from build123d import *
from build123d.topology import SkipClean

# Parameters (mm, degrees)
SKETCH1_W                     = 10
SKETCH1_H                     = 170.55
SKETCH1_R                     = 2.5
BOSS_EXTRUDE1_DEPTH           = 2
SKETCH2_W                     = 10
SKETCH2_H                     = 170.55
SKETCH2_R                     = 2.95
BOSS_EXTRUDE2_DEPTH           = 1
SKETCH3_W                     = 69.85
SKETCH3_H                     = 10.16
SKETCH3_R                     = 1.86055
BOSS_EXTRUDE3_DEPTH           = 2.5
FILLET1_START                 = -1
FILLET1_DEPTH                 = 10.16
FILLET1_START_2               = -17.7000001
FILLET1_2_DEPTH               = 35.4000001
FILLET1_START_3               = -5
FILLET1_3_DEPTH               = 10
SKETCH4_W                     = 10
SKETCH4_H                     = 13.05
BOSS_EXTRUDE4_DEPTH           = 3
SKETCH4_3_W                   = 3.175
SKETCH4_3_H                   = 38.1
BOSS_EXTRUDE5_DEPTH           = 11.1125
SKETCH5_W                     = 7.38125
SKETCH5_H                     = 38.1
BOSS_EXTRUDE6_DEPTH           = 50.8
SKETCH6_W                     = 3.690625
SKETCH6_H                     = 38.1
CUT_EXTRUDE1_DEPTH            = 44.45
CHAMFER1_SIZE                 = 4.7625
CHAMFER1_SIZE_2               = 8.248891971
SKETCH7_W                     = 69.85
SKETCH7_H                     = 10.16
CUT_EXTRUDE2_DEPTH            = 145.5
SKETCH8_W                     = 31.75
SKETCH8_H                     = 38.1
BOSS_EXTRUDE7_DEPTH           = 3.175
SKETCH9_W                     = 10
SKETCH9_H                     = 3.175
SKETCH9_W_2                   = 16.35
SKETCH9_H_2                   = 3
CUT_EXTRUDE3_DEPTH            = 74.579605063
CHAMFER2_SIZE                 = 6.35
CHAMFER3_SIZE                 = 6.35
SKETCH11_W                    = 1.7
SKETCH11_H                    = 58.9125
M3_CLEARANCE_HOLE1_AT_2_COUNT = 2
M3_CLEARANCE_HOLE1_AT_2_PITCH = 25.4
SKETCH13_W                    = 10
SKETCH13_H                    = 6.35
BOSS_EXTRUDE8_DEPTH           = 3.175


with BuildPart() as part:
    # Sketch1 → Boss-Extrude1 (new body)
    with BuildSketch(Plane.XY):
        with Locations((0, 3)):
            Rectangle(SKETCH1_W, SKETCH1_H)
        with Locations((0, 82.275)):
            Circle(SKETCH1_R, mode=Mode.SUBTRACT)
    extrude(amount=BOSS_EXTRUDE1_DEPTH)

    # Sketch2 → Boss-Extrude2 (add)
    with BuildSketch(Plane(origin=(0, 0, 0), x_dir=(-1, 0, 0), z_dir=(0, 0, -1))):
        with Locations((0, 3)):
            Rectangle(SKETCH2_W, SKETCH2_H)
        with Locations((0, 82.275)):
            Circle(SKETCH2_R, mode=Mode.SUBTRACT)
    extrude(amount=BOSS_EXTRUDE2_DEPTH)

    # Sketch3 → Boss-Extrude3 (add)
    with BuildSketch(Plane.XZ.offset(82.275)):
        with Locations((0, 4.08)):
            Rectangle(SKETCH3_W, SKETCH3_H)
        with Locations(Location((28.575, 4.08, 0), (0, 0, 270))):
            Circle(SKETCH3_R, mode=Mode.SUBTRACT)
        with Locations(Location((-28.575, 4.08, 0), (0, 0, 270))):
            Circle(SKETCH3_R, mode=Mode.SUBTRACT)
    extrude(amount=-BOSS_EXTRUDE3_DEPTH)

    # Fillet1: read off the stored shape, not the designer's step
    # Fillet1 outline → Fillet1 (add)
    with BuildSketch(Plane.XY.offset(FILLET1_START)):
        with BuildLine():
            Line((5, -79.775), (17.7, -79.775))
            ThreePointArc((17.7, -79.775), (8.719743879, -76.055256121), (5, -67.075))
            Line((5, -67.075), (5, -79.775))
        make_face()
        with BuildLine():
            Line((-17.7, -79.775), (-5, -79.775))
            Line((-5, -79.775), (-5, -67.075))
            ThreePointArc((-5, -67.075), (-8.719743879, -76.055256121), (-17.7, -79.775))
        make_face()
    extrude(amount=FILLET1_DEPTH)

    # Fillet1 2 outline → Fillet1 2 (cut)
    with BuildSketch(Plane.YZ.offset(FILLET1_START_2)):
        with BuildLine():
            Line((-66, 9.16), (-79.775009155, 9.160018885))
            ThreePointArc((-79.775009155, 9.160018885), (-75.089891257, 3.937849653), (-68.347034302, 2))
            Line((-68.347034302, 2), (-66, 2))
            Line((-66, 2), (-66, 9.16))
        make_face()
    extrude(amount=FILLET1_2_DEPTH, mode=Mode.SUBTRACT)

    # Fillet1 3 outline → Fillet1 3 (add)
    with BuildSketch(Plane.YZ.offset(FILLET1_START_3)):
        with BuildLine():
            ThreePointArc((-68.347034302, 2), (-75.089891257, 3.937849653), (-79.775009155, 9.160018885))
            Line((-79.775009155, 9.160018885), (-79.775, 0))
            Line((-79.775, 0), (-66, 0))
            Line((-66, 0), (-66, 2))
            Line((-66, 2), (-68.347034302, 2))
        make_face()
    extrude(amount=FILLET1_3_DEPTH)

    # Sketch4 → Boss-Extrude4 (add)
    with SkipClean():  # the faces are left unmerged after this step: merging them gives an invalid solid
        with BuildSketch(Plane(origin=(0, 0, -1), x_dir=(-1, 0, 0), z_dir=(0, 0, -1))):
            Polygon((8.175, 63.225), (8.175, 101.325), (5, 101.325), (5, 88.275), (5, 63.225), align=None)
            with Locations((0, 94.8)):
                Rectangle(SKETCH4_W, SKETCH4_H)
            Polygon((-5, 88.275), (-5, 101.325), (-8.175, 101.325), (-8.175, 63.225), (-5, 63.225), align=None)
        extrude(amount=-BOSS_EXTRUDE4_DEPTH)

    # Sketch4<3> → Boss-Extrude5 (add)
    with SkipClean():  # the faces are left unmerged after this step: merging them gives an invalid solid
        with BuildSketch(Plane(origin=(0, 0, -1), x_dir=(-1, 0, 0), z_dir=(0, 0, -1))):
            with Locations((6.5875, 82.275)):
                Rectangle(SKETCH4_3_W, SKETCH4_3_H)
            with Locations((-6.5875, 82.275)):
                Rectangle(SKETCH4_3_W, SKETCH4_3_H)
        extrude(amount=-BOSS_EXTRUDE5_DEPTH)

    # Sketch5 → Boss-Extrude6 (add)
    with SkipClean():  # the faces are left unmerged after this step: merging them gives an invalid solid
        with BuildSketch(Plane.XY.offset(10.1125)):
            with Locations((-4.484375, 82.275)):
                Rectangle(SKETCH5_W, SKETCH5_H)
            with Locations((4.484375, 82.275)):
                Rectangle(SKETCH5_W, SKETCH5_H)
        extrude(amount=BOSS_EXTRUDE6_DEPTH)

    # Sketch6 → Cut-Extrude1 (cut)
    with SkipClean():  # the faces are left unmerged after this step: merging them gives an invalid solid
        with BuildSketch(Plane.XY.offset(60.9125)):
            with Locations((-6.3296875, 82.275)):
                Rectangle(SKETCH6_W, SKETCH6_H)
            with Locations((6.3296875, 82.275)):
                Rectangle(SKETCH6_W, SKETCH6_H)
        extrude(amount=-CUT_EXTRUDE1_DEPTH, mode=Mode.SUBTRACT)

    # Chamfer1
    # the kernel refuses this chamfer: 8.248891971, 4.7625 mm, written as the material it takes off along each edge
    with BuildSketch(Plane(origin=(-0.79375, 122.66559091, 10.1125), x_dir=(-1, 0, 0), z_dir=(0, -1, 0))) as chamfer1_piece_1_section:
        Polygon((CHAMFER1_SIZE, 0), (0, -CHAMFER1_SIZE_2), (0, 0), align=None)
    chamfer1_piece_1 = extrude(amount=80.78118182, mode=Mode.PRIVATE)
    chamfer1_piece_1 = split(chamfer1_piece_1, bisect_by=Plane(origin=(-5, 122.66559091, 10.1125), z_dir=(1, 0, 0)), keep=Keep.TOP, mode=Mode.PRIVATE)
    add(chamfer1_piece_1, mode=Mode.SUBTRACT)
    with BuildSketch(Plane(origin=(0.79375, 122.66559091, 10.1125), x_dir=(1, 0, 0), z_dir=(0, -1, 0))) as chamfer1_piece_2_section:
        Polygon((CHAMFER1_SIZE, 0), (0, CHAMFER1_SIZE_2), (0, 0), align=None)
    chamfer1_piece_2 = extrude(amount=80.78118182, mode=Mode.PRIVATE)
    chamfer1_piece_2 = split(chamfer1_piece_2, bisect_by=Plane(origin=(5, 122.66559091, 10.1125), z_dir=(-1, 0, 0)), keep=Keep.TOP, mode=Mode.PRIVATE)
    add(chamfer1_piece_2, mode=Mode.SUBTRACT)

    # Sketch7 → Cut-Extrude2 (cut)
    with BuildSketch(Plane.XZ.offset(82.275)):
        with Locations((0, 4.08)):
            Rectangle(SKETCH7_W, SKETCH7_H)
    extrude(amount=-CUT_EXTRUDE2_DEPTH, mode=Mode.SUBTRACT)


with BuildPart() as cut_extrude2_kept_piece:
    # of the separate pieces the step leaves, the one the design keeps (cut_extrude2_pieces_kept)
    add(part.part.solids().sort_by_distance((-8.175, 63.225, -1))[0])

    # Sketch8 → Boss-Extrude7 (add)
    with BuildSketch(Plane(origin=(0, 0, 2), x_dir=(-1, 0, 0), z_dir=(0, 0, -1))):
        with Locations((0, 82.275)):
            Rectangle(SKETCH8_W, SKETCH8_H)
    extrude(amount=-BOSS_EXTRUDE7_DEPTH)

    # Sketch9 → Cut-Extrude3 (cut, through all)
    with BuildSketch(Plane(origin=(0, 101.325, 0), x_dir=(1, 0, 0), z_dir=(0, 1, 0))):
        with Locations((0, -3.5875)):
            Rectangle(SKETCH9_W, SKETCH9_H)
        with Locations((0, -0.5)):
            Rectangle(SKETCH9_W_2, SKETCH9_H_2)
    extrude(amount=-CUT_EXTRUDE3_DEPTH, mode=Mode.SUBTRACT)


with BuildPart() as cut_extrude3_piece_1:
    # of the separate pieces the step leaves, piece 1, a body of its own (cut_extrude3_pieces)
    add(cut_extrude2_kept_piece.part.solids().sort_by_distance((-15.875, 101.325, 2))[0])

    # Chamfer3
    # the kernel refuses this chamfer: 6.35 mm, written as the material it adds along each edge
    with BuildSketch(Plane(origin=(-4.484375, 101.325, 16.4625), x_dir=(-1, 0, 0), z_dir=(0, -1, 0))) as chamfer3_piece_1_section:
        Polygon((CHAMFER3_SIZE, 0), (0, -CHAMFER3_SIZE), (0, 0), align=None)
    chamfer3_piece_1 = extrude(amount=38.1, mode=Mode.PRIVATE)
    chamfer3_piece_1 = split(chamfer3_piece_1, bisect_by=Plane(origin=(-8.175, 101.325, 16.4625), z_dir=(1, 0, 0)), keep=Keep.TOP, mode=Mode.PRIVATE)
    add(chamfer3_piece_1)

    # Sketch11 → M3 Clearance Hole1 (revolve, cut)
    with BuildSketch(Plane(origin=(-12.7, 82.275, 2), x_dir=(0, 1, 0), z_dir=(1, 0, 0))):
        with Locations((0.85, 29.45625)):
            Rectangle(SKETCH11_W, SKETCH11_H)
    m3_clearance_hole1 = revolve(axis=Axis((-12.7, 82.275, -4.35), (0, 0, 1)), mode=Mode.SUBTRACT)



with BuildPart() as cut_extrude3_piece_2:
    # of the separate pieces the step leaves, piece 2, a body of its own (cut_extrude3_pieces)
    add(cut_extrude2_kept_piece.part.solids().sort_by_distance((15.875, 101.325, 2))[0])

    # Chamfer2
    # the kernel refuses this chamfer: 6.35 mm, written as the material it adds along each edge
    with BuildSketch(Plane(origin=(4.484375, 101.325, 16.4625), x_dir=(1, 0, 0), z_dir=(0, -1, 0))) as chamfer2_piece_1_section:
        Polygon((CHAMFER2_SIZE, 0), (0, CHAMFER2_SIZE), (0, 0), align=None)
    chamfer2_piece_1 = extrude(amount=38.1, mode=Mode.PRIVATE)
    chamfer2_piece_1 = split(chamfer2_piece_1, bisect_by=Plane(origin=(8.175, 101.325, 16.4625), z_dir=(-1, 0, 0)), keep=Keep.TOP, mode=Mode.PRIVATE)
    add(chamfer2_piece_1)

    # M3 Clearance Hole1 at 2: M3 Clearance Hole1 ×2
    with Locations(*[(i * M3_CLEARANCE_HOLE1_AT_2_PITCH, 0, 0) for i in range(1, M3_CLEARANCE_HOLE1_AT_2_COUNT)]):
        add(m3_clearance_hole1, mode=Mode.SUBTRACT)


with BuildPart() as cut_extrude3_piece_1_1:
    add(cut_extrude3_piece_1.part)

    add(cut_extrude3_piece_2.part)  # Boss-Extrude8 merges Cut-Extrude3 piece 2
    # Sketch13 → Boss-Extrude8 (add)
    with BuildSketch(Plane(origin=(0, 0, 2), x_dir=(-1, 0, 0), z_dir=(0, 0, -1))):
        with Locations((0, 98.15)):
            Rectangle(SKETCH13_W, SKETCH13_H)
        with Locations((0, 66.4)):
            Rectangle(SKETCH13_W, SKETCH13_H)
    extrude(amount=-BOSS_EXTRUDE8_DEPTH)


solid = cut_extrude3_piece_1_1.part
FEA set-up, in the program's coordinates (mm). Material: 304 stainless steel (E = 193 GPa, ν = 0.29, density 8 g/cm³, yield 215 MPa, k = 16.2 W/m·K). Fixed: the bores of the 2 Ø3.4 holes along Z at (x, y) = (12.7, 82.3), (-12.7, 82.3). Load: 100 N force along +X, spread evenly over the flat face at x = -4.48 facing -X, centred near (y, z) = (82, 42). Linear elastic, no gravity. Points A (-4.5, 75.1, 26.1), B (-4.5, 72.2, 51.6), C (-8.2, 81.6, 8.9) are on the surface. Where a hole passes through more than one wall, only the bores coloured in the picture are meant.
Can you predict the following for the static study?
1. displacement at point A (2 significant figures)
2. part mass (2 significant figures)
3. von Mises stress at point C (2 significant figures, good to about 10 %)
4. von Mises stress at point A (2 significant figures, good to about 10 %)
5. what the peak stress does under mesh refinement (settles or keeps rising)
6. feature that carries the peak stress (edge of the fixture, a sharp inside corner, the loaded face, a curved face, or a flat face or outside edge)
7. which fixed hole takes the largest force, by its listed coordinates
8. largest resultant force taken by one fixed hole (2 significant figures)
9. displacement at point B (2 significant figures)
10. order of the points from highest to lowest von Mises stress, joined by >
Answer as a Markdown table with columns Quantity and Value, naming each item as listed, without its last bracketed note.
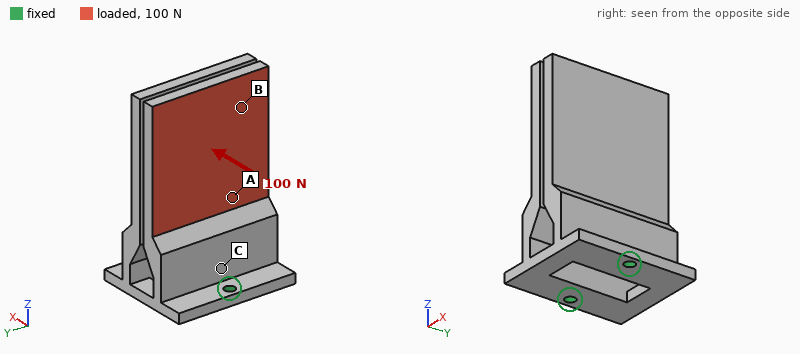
| Quantity | Value |
|---|---|
| displacement at point A | 0.049 mm |
| part mass | 160 g |
| von Mises stress at point C | 44 MPa |
| von Mises stress at point A | 18 MPa |
| what the peak stress does under mesh refinement | keeps rising |
| feature that carries the peak stress | edge of the fixture |
| which fixed hole takes the largest force, by its listed coordinates | (-12.7, 82.3) |
| largest resultant force taken by one fixed hole | 160 N |
| displacement at point B | 0.13 mm |
| order of the points from highest to lowest von Mises stress, joined by > | C > A > B |
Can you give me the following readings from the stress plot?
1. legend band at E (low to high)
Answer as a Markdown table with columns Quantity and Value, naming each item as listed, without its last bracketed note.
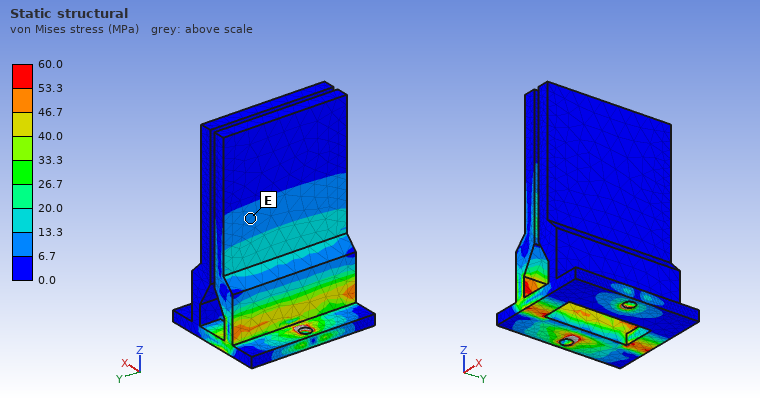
| Quantity | Value |
|---|---|
| legend band at E | 6.7 to 13.3 MPa |
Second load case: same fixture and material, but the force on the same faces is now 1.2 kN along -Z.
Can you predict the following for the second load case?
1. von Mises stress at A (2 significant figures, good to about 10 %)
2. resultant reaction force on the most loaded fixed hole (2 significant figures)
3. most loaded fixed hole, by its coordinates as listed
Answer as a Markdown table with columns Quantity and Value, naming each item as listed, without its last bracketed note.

| Quantity | Value |
|---|---|
| von Mises stress at A | 30 MPa |
| resultant reaction force on the most loaded fixed hole | 940 N |
| most loaded fixed hole, by its coordinates as listed | (-12.7, 82.3) |
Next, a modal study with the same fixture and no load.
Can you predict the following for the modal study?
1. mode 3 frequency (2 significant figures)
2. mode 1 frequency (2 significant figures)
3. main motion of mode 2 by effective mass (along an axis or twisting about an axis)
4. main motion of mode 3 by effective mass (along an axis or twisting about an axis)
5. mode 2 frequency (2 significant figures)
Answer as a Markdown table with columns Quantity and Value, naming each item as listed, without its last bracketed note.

| Quantity | Value |
|---|---|
| mode 3 frequency | 940 Hz |
| mode 1 frequency | 660 Hz |
| main motion of mode 2 by effective mass | along X |
| main motion of mode 3 by effective mass | along Y |
| mode 2 frequency | 780 Hz |
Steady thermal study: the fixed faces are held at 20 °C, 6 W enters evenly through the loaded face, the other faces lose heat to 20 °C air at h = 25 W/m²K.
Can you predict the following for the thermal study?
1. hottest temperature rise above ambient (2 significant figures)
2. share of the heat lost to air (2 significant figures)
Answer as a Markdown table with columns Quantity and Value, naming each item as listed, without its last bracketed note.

| Quantity | Value |
|---|---|
| hottest temperature rise above ambient | 61 K |
| share of the heat lost to air | 67 % |
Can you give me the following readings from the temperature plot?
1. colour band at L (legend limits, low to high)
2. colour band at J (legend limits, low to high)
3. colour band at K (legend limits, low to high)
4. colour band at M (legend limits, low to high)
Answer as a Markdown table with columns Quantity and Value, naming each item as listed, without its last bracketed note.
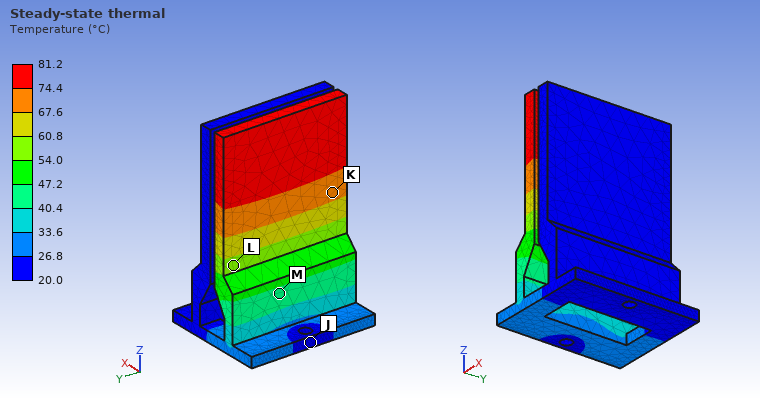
| Quantity | Value |
|---|---|
| colour band at L | 54.0 to 60.8 °C |
| colour band at J | 20.0 to 26.8 °C |
| colour band at K | 67.6 to 74.4 °C |
| colour band at M | 40.4 to 47.2 °C |
